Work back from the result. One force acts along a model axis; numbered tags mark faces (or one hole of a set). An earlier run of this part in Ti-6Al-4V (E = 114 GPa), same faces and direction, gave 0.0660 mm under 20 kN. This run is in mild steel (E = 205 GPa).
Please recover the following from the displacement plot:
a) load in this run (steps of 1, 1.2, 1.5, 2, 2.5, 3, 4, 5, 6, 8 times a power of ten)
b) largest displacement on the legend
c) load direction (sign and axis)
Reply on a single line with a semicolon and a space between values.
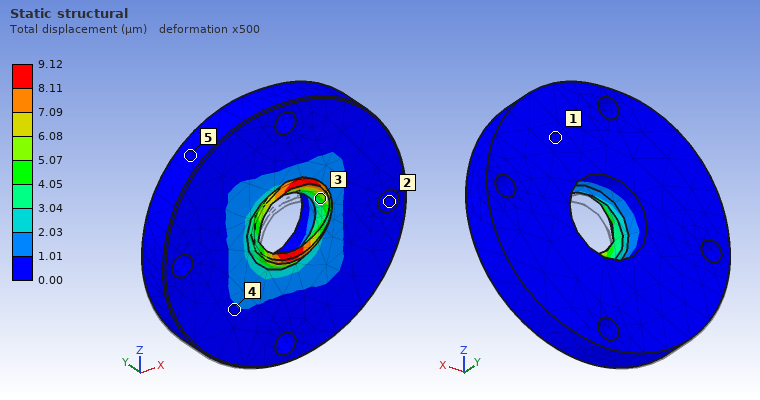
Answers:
5 kN; 9.12 µm; +Z
